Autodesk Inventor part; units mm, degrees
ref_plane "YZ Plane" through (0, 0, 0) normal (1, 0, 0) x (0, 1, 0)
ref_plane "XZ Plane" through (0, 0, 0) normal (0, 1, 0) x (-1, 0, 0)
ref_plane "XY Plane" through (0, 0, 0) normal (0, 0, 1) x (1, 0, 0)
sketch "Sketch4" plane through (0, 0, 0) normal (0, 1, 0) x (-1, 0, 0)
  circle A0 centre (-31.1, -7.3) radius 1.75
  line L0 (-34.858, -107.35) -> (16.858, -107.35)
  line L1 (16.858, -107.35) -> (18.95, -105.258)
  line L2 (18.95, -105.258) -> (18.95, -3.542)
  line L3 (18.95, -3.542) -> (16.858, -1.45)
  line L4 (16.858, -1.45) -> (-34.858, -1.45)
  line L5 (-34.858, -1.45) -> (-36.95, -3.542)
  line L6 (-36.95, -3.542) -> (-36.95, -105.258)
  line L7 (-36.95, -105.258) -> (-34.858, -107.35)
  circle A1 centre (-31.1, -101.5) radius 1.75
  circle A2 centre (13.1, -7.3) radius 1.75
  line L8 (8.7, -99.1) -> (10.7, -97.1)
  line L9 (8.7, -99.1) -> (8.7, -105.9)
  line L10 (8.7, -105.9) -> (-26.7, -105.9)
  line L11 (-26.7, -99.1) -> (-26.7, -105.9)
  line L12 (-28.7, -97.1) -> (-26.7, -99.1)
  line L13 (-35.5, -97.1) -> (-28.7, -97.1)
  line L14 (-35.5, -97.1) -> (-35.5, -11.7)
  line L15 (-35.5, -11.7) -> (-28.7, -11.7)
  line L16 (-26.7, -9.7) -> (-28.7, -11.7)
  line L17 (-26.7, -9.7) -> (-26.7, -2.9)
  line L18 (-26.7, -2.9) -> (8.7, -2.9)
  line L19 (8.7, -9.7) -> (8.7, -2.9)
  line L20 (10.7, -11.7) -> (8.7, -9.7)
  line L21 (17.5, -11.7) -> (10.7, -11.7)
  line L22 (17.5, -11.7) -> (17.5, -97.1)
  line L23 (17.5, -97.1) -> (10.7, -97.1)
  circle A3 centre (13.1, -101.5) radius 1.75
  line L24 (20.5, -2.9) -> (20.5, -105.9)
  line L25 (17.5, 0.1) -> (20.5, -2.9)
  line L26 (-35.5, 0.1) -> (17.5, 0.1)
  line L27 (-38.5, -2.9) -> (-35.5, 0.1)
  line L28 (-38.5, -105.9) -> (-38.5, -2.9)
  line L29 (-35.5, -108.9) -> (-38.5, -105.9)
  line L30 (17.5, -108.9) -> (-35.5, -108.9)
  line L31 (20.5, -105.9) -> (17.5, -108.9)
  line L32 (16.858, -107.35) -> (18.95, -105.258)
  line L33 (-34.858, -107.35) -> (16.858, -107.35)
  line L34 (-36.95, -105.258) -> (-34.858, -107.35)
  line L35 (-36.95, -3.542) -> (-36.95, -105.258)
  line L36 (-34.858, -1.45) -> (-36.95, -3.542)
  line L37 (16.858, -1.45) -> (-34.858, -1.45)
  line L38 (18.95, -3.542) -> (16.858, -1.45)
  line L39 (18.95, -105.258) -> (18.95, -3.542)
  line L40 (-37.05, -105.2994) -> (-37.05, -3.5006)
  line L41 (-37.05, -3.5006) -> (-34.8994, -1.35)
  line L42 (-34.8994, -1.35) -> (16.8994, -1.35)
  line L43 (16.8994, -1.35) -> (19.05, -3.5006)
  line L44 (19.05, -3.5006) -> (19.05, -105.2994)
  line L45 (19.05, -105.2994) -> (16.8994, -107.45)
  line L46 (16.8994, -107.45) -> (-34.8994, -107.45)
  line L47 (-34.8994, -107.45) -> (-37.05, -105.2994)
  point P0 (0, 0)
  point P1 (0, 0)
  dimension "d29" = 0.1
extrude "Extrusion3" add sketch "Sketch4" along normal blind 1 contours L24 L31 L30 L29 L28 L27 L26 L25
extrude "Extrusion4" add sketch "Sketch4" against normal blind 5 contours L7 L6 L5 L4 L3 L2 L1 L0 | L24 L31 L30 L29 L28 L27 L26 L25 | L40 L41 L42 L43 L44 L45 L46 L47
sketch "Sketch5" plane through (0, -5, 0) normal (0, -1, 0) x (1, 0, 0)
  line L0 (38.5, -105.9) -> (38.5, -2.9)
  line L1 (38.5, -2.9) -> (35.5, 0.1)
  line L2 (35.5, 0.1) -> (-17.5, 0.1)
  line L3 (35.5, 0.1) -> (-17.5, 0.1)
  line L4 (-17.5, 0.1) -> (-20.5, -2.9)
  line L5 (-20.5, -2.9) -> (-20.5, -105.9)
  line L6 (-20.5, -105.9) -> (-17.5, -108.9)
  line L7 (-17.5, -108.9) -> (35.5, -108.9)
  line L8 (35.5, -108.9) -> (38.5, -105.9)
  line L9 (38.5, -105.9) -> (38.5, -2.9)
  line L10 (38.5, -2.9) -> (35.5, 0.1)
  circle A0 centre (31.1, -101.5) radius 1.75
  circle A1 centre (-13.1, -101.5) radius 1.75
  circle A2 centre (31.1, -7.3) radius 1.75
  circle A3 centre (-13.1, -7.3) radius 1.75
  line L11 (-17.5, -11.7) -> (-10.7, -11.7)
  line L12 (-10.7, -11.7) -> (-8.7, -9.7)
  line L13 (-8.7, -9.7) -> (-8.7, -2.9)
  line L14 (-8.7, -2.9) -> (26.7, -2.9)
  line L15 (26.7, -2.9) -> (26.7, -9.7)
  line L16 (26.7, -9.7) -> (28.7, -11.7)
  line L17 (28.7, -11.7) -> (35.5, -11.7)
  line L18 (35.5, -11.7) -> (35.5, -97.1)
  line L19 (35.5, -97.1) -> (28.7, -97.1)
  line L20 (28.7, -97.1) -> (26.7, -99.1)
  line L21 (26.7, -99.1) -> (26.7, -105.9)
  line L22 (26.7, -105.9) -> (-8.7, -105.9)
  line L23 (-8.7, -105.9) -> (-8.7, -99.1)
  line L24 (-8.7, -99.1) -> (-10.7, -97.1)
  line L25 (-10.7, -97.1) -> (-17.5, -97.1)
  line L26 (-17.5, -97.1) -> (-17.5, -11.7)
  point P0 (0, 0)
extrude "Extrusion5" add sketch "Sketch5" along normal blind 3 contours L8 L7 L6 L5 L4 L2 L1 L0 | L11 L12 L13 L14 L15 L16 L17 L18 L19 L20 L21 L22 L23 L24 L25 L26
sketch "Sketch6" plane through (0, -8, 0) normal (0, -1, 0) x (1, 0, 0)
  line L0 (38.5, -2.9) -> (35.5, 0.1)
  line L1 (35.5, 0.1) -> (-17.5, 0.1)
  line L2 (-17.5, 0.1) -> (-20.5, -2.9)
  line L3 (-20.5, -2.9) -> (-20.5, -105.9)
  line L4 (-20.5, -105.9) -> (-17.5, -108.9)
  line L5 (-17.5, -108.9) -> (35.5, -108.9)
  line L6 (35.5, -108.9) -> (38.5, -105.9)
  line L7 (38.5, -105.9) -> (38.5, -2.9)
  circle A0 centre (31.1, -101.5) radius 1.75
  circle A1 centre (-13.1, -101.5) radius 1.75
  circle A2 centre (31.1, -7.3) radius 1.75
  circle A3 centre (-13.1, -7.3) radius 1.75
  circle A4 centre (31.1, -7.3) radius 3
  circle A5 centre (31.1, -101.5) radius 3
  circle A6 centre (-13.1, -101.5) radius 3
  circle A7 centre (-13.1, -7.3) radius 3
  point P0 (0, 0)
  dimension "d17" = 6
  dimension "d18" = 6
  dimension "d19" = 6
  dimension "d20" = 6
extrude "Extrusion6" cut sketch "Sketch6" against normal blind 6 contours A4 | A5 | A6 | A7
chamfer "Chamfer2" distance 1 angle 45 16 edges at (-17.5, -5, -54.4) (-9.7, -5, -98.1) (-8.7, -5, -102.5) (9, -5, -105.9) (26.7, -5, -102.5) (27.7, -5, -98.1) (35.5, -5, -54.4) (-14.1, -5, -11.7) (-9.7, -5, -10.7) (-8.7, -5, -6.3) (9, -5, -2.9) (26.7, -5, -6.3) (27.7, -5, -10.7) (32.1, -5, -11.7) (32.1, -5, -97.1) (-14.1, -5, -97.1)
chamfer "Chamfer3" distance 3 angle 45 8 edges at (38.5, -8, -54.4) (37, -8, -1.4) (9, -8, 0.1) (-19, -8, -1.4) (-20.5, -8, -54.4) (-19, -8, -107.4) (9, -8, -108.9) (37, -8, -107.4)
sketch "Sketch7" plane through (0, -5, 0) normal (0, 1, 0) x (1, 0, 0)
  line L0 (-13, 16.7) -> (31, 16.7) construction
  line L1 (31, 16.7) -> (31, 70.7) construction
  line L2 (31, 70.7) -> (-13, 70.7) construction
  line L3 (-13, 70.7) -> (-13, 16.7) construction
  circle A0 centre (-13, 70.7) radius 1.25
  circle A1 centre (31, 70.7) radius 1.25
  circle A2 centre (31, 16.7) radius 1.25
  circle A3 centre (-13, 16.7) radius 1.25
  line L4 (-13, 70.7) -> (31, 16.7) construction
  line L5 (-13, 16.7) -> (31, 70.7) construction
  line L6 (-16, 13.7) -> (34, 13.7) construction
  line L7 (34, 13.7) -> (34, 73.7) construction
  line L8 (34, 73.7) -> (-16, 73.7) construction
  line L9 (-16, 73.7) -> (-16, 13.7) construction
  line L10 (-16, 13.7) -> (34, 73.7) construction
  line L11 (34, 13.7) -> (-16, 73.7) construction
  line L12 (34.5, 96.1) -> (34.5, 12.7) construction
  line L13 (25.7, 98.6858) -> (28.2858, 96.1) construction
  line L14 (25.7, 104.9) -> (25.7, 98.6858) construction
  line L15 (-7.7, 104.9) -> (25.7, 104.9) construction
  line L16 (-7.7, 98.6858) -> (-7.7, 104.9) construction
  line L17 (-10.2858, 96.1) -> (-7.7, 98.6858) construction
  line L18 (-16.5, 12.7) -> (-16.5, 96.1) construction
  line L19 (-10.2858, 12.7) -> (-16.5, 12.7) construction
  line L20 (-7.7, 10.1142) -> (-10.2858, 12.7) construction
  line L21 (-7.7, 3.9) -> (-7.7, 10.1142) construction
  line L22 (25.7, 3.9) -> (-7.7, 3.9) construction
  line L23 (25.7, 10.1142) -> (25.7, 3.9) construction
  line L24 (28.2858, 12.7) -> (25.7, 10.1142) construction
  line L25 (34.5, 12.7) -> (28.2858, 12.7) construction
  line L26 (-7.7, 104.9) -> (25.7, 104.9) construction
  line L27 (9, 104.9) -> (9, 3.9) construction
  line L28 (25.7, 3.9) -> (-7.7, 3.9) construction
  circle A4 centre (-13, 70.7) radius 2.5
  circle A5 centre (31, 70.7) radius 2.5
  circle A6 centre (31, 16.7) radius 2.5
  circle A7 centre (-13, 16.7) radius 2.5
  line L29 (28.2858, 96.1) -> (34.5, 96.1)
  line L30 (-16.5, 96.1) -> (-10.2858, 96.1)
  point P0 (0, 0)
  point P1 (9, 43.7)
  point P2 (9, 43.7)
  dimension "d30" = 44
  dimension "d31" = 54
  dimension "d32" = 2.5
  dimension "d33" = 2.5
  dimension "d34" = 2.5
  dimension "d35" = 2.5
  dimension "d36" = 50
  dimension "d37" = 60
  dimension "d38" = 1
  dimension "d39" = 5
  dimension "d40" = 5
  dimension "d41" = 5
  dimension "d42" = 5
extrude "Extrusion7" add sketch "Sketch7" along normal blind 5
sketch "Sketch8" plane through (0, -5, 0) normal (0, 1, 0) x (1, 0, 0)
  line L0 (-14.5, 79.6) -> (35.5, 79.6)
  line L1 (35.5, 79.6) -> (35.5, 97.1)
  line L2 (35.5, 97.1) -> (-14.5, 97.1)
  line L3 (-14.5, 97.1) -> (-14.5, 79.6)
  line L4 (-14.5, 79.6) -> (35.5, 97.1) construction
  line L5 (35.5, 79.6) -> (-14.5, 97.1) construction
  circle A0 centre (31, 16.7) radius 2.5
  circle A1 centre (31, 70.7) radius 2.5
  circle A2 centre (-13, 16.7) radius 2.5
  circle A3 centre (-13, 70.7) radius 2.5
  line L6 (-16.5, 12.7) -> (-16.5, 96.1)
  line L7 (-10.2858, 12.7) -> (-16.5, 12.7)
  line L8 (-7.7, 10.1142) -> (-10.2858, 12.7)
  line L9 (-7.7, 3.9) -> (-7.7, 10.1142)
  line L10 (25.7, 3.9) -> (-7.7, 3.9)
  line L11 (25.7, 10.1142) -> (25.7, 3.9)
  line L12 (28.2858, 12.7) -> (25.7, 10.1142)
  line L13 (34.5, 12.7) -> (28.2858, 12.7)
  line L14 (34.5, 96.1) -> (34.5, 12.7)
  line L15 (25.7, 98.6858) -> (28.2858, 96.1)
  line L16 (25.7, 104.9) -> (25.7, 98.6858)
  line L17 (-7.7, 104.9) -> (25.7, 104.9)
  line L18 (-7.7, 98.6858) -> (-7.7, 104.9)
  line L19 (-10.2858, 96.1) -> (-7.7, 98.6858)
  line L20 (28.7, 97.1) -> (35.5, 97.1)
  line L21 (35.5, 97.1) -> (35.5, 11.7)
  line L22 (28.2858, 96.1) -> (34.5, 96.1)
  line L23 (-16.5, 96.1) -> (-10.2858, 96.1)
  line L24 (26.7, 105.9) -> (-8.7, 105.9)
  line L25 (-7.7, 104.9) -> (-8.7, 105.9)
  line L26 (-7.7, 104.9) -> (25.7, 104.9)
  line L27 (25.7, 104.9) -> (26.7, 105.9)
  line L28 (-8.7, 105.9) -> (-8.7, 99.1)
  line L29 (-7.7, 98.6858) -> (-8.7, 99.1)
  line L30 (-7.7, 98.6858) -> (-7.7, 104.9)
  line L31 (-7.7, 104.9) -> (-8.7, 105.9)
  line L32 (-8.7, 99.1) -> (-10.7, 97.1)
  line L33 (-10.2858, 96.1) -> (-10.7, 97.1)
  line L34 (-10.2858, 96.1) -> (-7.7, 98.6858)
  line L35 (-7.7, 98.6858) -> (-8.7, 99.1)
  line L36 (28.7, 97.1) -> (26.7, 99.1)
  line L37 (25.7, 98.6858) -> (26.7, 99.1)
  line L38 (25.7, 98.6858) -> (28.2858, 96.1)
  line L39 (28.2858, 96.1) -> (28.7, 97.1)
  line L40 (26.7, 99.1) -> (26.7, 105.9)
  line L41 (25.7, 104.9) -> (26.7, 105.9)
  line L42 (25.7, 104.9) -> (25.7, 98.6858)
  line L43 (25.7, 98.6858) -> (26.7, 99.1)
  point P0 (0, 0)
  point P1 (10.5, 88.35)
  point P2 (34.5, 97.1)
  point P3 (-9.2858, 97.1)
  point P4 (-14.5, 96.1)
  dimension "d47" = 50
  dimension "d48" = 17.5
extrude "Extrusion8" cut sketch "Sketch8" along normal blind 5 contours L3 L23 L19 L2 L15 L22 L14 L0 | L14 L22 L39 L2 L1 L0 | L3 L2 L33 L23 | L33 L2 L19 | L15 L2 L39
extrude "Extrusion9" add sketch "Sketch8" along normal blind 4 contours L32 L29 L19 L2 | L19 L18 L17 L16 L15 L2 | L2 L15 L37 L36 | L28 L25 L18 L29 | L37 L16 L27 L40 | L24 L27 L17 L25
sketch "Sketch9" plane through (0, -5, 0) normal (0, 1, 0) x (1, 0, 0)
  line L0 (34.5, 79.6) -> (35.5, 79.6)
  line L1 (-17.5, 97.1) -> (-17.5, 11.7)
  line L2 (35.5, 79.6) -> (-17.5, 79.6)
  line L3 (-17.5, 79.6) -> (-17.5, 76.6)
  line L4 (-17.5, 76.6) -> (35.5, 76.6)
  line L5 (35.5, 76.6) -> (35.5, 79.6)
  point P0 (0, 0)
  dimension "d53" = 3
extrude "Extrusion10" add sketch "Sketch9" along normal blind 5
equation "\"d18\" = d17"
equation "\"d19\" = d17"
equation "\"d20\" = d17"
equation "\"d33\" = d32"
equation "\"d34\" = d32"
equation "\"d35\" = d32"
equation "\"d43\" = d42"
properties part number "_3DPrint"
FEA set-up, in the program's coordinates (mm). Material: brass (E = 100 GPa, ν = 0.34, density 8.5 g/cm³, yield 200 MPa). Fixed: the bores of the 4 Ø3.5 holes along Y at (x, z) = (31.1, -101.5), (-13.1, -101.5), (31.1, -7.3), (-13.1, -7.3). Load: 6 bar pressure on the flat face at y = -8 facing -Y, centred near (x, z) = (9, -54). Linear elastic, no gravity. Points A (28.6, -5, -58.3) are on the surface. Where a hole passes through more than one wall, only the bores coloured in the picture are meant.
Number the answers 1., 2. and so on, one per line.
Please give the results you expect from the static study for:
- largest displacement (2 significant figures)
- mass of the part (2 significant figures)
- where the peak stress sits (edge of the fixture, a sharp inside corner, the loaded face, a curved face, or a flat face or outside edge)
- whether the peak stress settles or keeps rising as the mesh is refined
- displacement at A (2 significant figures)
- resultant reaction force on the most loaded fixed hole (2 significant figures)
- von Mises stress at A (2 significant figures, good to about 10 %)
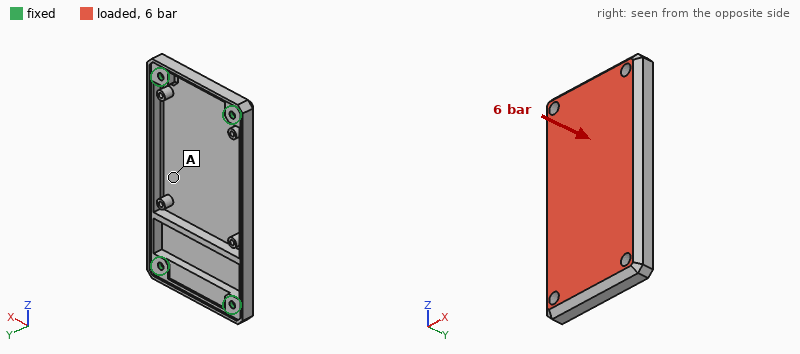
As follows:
1. 0.23 mm
2. 220 g
3. edge of the fixture
4. keeps rising
5. 0.18 mm
6. 1.7 kN
7. 27 MPa
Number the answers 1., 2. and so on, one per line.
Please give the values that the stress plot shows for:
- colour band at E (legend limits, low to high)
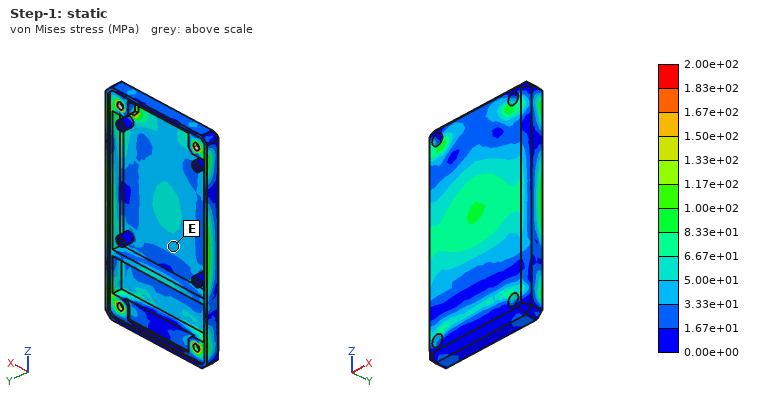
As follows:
1. 3.33e+01 to 5.00e+01 MPa
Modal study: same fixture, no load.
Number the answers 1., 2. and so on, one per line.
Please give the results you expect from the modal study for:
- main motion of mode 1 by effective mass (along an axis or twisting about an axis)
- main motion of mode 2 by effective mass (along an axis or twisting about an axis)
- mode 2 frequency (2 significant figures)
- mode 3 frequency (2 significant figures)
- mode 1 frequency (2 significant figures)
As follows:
1. along Y
2. twisting about Z
3. 2500 Hz
4. 3700 Hz
5. 1800 Hz
